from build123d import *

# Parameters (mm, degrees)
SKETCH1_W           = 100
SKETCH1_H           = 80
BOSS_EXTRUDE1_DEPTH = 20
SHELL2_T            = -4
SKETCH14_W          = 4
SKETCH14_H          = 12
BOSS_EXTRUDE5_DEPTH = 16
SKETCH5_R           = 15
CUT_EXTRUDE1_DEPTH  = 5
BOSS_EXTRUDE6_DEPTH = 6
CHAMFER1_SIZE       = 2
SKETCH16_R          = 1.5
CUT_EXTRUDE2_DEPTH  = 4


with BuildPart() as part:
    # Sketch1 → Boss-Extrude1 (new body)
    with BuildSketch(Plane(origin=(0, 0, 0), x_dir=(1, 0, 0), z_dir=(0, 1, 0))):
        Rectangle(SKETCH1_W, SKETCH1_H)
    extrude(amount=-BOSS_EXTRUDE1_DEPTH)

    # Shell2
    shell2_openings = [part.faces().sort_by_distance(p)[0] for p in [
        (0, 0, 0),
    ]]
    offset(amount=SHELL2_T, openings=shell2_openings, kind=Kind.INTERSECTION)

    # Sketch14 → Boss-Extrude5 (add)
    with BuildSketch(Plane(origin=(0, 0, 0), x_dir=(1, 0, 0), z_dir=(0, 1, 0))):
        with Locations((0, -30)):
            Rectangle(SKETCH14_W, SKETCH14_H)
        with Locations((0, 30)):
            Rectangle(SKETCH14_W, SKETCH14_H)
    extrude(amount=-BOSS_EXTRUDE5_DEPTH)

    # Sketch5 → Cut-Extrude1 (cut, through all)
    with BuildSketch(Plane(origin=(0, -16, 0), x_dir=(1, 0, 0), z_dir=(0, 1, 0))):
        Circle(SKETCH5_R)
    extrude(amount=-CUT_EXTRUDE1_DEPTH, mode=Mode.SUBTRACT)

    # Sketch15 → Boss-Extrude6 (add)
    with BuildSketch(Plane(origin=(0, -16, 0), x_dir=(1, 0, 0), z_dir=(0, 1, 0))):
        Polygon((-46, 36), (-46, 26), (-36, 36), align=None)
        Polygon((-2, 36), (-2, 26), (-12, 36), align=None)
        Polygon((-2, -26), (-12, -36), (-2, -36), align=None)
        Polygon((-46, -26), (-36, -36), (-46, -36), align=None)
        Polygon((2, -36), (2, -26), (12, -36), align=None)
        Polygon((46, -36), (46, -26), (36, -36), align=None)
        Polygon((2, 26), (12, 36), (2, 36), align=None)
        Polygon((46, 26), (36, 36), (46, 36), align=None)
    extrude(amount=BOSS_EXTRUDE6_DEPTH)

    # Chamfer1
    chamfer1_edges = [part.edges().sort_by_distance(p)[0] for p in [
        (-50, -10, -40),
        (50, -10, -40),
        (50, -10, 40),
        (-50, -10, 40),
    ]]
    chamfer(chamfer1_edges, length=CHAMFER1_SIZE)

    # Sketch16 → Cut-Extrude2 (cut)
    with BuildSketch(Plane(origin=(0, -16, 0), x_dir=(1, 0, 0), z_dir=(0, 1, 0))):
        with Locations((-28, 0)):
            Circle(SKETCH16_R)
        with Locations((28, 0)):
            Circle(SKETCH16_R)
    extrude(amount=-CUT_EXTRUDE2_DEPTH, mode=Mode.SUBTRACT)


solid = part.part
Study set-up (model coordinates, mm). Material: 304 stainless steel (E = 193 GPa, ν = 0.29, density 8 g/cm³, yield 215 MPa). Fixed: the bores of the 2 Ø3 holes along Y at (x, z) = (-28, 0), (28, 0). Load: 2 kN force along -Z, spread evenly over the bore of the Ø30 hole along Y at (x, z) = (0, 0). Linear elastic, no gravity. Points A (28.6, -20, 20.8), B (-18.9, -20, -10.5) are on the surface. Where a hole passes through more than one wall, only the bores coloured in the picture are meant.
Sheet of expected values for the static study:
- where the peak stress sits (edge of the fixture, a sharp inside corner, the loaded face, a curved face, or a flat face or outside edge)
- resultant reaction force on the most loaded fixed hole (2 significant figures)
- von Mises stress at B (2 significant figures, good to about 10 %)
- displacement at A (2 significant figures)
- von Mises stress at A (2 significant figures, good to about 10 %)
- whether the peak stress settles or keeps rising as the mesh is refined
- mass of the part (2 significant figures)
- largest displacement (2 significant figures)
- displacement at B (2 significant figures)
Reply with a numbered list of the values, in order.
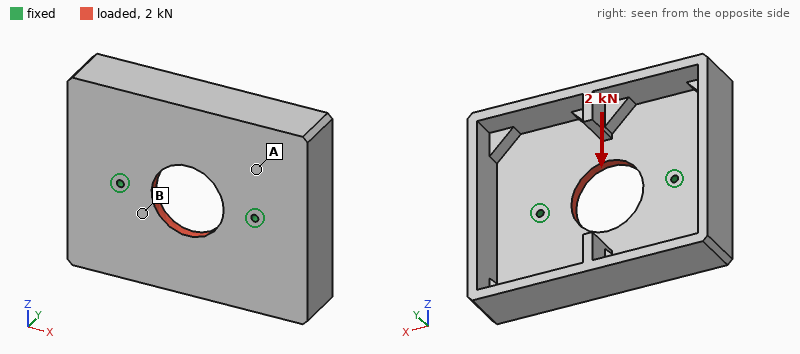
1. edge of the fixture
2. 1.0 kN
3. 7.4 MPa
4. 0.79 µm
5. 3.3 MPa
6. keeps rising
7. 440 g
8. 1.9 µm
9. 1.1 µm
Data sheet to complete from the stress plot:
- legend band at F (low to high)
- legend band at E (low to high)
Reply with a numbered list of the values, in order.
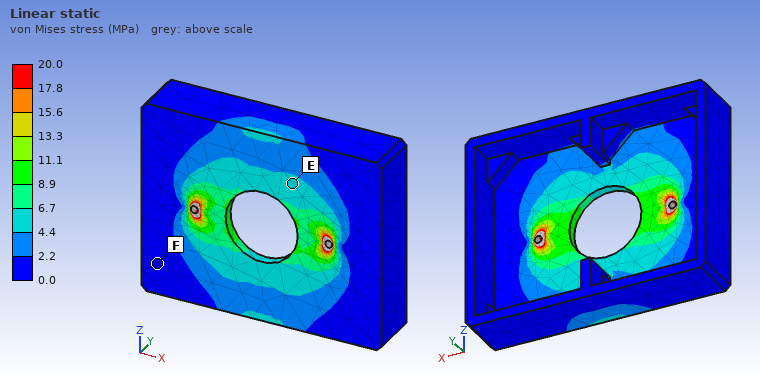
1. 0.0 to 2.2 MPa
2. 4.4 to 6.7 MPa
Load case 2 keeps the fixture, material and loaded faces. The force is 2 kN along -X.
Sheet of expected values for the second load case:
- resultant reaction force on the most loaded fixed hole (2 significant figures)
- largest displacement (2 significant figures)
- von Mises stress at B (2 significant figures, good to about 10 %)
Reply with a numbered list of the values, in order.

1. 1.0 kN
2. 1.7 µm
3. 7.0 MPa
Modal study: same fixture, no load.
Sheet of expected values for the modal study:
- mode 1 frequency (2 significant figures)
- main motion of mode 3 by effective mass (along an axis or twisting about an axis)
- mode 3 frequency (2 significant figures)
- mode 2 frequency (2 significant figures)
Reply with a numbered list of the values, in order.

1. 780 Hz
2. along Y
3. 2100 Hz
4. 1600 Hz
